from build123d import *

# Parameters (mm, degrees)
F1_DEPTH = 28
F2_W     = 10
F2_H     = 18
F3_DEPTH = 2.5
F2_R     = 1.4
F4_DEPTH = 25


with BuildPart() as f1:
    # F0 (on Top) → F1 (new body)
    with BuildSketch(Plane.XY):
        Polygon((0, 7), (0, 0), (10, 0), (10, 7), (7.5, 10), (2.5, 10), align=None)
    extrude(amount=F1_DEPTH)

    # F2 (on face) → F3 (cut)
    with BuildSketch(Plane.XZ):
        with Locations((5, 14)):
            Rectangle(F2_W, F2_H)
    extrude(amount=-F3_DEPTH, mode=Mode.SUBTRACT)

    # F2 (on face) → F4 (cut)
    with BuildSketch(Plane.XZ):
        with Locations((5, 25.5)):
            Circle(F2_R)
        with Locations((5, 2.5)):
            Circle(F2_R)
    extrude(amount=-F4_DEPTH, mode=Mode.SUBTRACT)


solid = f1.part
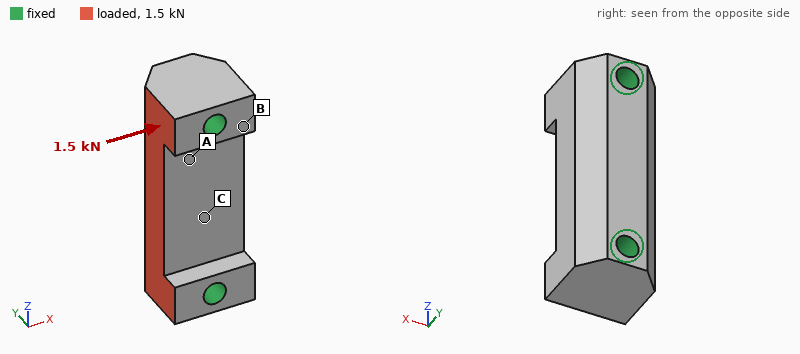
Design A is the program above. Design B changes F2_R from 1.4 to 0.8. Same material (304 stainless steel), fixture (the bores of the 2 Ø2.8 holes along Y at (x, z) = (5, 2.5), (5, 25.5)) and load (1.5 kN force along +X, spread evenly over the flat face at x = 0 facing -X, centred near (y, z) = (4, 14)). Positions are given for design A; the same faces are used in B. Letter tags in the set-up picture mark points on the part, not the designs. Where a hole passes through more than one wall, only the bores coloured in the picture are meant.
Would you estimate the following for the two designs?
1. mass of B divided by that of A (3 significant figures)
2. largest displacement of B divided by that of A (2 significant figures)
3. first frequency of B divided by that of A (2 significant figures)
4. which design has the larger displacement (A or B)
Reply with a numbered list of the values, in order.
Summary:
1. 1.04
2. 1.3
3. 0.83
4. B
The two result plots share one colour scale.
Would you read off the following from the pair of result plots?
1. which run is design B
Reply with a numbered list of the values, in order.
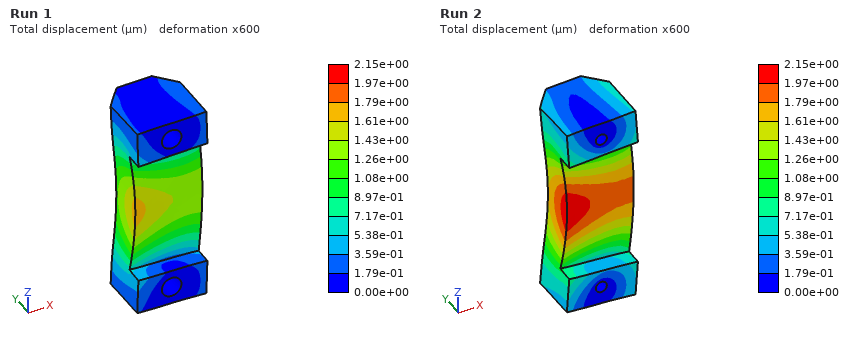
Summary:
1. Run 2
